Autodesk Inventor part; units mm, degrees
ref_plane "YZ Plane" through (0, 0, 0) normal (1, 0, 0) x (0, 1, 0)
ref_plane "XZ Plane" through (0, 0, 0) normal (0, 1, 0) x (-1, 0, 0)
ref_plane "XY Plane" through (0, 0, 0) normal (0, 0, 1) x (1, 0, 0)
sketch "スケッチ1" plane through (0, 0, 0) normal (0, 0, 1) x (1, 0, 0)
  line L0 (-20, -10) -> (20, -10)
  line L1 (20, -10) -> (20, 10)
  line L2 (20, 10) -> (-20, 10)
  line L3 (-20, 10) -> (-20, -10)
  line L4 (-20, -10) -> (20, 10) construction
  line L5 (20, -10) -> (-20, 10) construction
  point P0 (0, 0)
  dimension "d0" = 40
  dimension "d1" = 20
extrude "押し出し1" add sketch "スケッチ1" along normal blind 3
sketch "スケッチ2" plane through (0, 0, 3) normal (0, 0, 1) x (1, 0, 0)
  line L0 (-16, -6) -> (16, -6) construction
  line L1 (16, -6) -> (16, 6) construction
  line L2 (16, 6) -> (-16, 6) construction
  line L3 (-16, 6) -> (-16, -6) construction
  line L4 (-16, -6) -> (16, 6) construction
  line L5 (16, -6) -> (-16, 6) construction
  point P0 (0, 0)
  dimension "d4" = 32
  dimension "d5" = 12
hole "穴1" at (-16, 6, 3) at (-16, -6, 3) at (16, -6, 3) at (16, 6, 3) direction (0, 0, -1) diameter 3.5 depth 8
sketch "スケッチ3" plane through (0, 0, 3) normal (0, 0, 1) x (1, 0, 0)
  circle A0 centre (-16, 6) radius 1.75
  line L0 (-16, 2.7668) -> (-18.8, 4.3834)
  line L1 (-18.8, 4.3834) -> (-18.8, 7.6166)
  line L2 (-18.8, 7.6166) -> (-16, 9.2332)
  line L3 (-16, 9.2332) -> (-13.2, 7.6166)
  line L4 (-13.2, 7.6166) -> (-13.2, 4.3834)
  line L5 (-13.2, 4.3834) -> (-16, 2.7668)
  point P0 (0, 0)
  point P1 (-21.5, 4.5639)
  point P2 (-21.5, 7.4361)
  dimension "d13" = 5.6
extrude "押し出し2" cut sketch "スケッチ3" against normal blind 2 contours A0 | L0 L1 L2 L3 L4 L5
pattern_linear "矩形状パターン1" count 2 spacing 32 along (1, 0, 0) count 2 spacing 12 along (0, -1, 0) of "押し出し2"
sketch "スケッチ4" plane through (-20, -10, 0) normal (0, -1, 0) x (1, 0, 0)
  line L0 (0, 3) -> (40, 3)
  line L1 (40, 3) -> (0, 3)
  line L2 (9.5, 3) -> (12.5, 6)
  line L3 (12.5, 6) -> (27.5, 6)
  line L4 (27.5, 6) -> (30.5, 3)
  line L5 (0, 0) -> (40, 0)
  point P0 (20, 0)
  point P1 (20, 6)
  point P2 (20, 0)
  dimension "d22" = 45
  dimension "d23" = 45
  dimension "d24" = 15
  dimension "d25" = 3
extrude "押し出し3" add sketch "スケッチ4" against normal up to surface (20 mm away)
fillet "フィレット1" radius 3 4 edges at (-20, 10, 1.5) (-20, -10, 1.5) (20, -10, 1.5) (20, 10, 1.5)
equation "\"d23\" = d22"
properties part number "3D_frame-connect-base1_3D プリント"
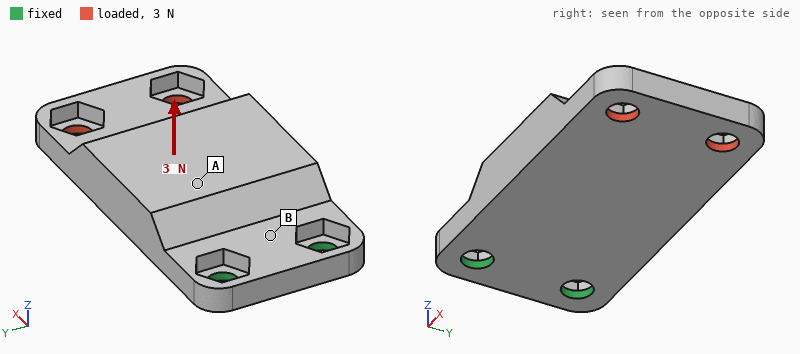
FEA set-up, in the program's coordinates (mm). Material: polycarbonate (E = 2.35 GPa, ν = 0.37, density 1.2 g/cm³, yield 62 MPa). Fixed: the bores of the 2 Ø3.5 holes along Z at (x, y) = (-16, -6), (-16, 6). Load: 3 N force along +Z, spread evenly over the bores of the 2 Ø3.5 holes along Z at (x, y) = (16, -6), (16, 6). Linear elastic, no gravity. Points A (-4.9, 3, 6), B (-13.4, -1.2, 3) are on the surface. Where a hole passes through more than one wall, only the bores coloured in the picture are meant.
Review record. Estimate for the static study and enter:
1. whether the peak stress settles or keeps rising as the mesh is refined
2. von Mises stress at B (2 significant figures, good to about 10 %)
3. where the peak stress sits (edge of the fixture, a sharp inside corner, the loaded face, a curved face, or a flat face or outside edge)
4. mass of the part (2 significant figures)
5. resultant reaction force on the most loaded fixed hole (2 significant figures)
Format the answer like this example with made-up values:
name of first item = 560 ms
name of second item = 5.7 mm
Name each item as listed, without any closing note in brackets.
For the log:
whether the peak stress settles or keeps rising as the mesh is refined = keeps rising
von Mises stress at B = 3.8 MPa
where the peak stress sits = edge of the fixture
mass of the part = 3.8 g
resultant reaction force on the most loaded fixed hole = 1.9 N
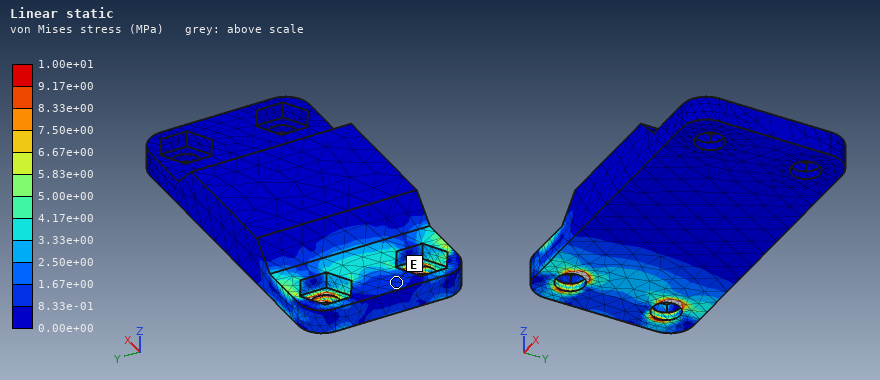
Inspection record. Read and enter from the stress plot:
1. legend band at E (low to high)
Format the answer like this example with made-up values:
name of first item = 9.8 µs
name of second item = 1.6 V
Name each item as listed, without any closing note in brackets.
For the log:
legend band at E = 8.33e-01 to 1.67e+00 MPa
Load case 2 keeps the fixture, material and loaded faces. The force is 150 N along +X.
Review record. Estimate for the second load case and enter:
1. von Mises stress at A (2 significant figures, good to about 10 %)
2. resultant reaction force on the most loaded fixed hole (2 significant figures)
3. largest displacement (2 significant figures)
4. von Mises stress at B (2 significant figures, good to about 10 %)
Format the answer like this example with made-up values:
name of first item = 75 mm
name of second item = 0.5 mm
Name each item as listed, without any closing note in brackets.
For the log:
von Mises stress at A = 1.8 MPa
resultant reaction force on the most loaded fixed hole = 76 N
largest displacement = 0.44 mm
von Mises stress at B = 1.7 MPa
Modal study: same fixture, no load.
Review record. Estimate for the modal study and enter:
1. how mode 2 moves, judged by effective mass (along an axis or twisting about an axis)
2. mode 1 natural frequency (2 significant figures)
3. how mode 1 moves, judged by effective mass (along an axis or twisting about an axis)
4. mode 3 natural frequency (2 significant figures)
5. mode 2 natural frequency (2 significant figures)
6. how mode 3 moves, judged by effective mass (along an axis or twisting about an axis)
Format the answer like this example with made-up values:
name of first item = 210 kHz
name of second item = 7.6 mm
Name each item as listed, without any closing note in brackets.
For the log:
how mode 2 moves, judged by effective mass = along Y
mode 1 natural frequency = 420 Hz
how mode 1 moves, judged by effective mass = along Z
mode 3 natural frequency = 2900 Hz
mode 2 natural frequency = 2100 Hz
how mode 3 moves, judged by effective mass = along Y
